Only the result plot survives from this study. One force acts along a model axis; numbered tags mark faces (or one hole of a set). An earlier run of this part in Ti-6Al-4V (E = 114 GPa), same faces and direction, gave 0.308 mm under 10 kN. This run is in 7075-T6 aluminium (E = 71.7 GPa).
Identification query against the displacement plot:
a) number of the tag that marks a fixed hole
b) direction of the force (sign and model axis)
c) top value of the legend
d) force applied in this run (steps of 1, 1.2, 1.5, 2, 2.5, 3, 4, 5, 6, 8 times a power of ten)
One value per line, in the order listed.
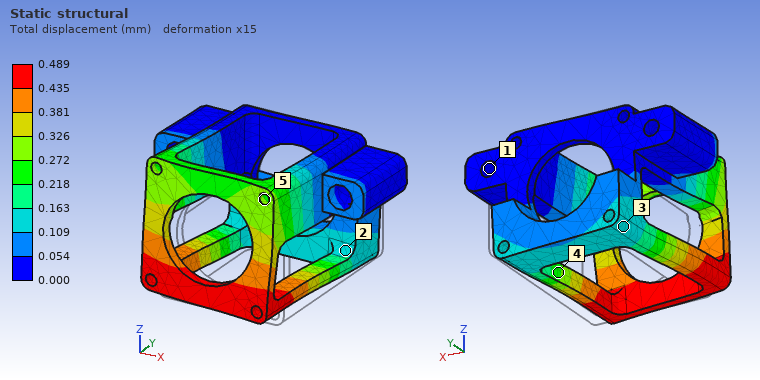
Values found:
1
-X
0.489 mm
10 kN
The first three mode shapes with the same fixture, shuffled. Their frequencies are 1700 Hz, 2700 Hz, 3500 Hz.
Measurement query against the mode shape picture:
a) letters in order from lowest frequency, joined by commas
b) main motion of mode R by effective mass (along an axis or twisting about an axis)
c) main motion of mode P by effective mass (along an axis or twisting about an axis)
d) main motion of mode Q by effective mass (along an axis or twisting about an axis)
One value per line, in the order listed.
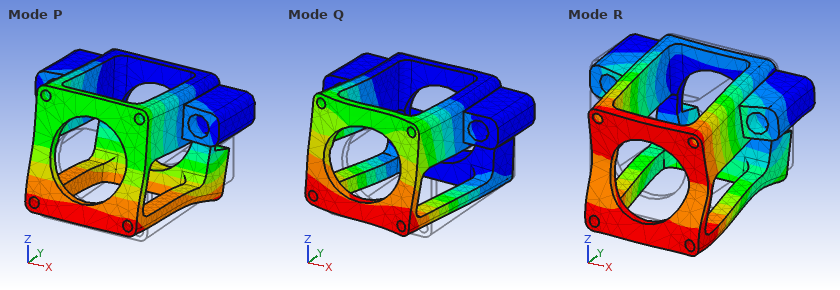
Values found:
P, Q, R
along Z
along Y
along X
